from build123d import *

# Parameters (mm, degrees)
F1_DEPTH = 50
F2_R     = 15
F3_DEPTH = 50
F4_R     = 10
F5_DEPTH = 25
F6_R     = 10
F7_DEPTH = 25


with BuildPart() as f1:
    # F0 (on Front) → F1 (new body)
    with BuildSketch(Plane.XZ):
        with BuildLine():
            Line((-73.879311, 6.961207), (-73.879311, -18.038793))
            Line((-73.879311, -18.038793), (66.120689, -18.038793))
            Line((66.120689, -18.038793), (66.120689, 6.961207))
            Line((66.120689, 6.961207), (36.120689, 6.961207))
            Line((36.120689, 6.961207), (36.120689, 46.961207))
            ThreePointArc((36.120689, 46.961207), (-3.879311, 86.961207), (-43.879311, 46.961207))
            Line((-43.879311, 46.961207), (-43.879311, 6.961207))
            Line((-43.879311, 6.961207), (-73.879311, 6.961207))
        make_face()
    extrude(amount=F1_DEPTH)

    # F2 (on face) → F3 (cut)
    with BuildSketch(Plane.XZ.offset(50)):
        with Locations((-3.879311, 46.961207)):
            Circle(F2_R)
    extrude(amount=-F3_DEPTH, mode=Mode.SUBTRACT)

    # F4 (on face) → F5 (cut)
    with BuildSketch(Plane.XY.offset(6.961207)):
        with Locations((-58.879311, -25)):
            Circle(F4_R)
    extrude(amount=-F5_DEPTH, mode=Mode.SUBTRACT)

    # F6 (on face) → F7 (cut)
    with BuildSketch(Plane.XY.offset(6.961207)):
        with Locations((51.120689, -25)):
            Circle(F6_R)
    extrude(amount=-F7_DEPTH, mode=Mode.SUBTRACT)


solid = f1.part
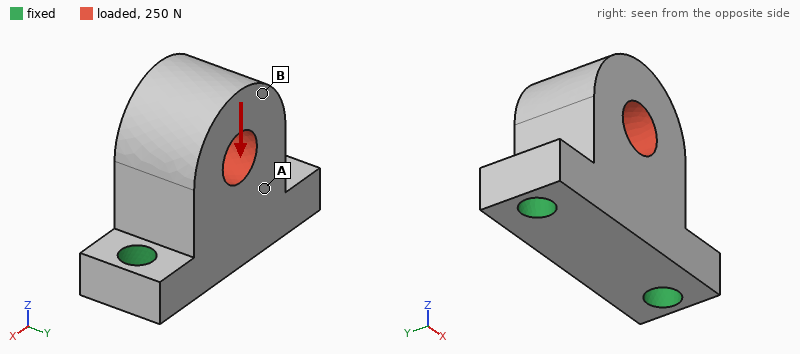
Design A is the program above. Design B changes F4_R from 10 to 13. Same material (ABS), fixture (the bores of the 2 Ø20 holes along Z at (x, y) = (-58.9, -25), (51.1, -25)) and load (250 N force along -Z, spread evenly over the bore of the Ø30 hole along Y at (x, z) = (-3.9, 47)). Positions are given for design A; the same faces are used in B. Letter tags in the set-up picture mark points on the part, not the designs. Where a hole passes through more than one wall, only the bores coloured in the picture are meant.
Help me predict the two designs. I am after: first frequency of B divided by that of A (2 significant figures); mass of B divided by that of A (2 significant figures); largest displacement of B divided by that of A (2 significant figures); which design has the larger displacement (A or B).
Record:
1.1
0.99
0.92
A
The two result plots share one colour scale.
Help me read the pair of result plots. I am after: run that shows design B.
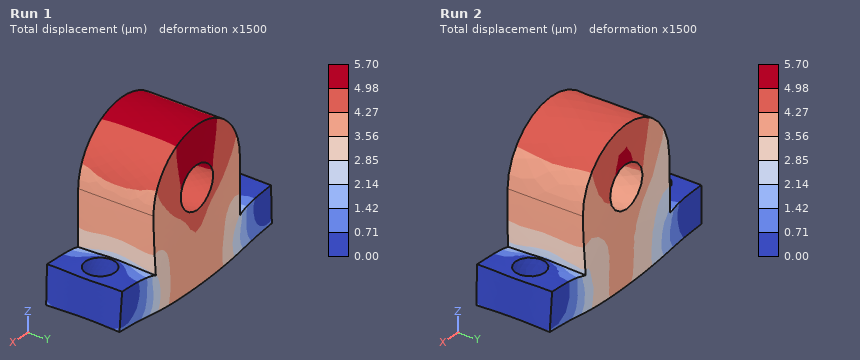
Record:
Run 2
